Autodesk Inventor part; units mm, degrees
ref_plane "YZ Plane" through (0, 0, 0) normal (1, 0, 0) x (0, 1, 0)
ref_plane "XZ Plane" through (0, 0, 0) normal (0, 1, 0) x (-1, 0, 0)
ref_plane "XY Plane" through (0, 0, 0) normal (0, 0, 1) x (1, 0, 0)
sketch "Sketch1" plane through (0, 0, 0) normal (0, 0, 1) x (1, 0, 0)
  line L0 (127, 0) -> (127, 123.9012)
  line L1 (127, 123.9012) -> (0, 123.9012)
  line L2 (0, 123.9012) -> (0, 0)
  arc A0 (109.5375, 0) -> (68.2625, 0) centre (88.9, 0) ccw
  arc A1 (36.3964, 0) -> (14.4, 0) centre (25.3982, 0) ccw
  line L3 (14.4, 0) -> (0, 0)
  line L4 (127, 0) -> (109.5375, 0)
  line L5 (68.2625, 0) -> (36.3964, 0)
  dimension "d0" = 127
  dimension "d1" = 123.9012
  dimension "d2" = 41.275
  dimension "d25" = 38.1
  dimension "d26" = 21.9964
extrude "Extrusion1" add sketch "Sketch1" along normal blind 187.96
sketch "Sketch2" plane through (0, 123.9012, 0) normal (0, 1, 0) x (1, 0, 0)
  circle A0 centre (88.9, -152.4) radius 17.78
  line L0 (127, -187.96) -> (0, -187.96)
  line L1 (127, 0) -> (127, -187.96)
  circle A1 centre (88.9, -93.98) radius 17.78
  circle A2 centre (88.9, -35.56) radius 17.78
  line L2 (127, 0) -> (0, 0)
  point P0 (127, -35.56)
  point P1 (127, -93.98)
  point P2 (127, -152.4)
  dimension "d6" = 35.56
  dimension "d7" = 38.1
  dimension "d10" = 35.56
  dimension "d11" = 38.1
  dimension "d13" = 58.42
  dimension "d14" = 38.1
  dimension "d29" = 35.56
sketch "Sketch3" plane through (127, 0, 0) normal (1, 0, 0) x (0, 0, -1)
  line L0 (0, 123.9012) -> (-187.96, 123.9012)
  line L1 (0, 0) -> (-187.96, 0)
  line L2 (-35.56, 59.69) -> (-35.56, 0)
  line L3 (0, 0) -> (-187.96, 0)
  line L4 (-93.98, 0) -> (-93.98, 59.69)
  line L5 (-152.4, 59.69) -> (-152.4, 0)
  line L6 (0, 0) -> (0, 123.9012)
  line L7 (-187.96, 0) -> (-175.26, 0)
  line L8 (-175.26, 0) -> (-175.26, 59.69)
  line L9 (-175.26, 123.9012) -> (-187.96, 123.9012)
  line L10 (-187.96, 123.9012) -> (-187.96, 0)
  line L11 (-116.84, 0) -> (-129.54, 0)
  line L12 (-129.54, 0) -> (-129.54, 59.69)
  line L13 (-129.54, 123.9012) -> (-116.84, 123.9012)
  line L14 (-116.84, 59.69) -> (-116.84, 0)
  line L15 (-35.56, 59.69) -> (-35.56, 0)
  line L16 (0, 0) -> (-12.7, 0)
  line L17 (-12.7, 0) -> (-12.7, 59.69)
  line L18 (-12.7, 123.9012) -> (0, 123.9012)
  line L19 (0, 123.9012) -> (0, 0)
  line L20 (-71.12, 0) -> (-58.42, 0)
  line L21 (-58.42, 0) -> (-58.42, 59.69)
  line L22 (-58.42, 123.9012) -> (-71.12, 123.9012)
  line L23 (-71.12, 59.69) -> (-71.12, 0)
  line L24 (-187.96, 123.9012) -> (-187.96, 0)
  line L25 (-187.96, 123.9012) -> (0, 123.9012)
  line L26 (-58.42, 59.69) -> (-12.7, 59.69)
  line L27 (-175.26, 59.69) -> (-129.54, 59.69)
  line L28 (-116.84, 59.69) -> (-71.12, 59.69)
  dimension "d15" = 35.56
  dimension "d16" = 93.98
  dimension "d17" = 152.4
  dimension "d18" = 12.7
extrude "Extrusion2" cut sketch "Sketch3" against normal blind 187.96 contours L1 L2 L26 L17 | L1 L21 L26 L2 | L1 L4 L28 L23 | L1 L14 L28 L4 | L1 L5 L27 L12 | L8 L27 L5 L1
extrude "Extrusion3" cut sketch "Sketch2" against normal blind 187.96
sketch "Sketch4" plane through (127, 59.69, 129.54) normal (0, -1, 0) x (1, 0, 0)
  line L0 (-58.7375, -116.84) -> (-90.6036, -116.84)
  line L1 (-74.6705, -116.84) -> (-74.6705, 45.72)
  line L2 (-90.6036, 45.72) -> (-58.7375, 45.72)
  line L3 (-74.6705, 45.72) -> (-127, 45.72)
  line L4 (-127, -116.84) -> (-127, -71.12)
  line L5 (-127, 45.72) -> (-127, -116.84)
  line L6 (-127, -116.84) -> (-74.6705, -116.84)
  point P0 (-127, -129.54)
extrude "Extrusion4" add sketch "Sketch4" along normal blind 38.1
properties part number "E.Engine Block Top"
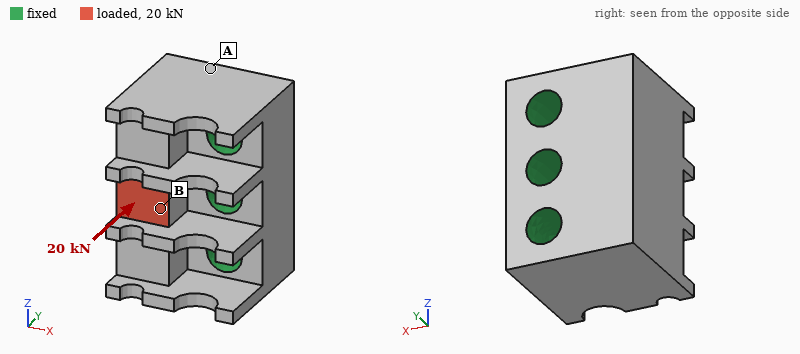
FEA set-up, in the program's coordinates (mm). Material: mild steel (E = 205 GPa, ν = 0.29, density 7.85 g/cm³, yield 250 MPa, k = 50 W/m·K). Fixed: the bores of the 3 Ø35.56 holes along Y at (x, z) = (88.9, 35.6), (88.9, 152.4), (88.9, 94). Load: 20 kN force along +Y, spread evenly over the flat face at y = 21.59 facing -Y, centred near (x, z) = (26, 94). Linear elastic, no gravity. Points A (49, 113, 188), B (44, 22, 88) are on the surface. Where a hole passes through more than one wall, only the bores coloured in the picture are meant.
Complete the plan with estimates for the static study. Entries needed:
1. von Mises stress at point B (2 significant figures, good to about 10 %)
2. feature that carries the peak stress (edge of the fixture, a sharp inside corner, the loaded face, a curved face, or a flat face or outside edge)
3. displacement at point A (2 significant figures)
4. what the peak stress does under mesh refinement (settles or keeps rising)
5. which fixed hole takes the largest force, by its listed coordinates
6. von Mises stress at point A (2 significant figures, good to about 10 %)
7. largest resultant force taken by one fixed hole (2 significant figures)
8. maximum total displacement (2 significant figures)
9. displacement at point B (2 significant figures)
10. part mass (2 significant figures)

7.9 MPa
edge of the fixture
0.91 µm
keeps rising
(88.9, 94)
1.5 MPa
8.4 kN
5.6 µm
3.7 µm
15 kg
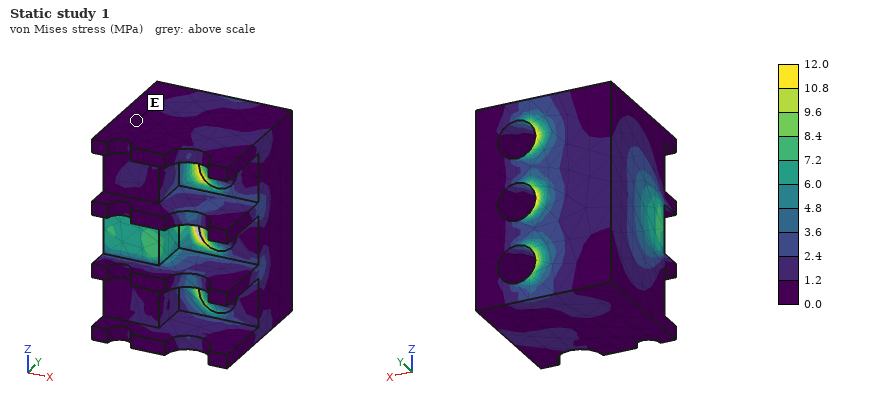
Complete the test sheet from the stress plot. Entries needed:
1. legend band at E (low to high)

0.0 to 1.2 MPa
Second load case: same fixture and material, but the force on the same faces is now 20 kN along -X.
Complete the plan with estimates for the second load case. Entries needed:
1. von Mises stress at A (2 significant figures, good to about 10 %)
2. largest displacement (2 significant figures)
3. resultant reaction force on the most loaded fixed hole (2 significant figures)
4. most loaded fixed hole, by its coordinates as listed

2.3 MPa
11 µm
10 kN
(88.9, 94)
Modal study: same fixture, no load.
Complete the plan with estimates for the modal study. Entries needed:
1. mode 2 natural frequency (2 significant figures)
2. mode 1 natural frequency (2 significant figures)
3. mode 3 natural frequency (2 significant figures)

3700 Hz
3700 Hz
4000 Hz
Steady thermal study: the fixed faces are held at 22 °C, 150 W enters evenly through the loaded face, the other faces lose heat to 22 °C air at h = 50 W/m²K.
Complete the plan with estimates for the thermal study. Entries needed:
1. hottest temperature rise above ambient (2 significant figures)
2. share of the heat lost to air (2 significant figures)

41 K
26 %
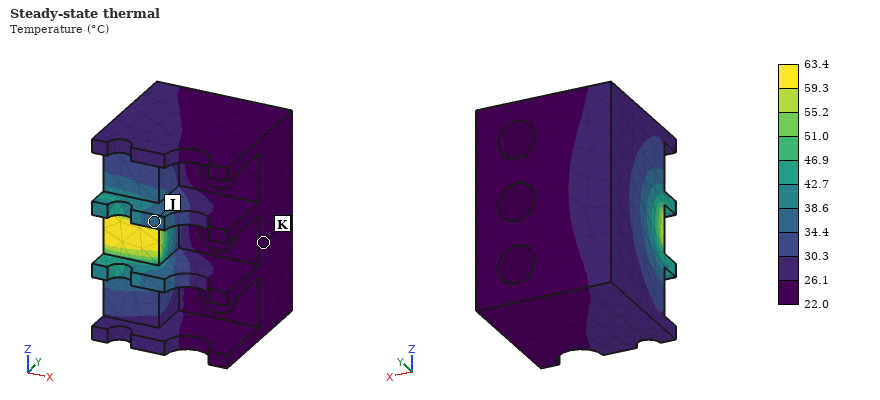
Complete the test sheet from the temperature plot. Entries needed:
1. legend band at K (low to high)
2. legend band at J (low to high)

22.0 to 26.1 °C
34.4 to 38.6 °C
